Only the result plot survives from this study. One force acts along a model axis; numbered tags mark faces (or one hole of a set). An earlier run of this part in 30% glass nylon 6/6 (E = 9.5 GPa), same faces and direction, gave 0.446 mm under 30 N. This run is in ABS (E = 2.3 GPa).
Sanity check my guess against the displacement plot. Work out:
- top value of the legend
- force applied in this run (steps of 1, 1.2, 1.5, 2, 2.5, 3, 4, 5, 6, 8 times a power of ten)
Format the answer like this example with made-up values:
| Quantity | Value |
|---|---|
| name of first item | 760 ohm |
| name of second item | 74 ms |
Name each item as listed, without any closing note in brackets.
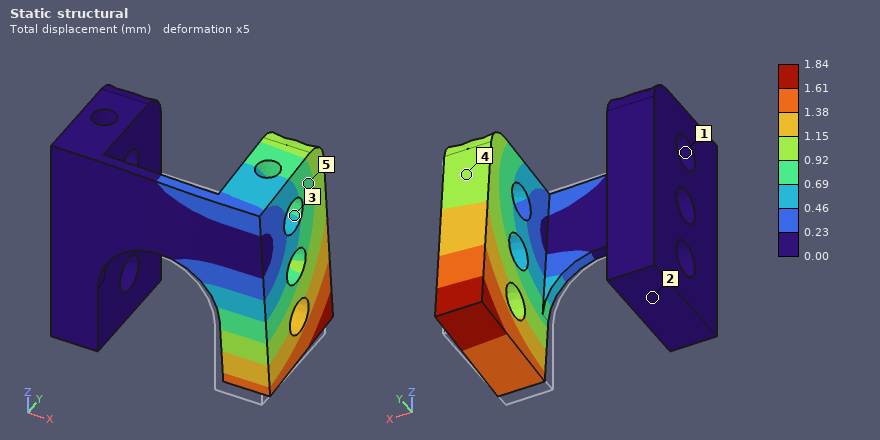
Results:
| Quantity | Value |
|---|---|
| top value of the legend | 1.84 mm |
| force applied in this run | 30 N |
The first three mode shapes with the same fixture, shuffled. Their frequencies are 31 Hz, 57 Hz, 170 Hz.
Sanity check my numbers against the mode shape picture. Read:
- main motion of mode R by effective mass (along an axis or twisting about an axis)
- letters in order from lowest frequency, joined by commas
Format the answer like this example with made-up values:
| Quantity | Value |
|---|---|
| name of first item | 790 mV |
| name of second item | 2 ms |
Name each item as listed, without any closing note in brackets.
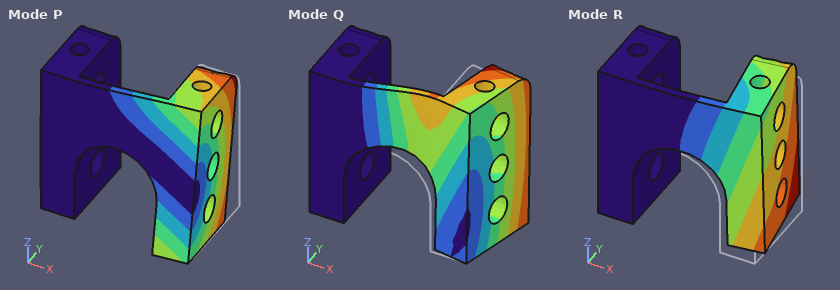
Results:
| Quantity | Value |
|---|---|
| main motion of mode R by effective mass | along Y |
| letters in order from lowest frequency, joined by commas | R, P, Q |
